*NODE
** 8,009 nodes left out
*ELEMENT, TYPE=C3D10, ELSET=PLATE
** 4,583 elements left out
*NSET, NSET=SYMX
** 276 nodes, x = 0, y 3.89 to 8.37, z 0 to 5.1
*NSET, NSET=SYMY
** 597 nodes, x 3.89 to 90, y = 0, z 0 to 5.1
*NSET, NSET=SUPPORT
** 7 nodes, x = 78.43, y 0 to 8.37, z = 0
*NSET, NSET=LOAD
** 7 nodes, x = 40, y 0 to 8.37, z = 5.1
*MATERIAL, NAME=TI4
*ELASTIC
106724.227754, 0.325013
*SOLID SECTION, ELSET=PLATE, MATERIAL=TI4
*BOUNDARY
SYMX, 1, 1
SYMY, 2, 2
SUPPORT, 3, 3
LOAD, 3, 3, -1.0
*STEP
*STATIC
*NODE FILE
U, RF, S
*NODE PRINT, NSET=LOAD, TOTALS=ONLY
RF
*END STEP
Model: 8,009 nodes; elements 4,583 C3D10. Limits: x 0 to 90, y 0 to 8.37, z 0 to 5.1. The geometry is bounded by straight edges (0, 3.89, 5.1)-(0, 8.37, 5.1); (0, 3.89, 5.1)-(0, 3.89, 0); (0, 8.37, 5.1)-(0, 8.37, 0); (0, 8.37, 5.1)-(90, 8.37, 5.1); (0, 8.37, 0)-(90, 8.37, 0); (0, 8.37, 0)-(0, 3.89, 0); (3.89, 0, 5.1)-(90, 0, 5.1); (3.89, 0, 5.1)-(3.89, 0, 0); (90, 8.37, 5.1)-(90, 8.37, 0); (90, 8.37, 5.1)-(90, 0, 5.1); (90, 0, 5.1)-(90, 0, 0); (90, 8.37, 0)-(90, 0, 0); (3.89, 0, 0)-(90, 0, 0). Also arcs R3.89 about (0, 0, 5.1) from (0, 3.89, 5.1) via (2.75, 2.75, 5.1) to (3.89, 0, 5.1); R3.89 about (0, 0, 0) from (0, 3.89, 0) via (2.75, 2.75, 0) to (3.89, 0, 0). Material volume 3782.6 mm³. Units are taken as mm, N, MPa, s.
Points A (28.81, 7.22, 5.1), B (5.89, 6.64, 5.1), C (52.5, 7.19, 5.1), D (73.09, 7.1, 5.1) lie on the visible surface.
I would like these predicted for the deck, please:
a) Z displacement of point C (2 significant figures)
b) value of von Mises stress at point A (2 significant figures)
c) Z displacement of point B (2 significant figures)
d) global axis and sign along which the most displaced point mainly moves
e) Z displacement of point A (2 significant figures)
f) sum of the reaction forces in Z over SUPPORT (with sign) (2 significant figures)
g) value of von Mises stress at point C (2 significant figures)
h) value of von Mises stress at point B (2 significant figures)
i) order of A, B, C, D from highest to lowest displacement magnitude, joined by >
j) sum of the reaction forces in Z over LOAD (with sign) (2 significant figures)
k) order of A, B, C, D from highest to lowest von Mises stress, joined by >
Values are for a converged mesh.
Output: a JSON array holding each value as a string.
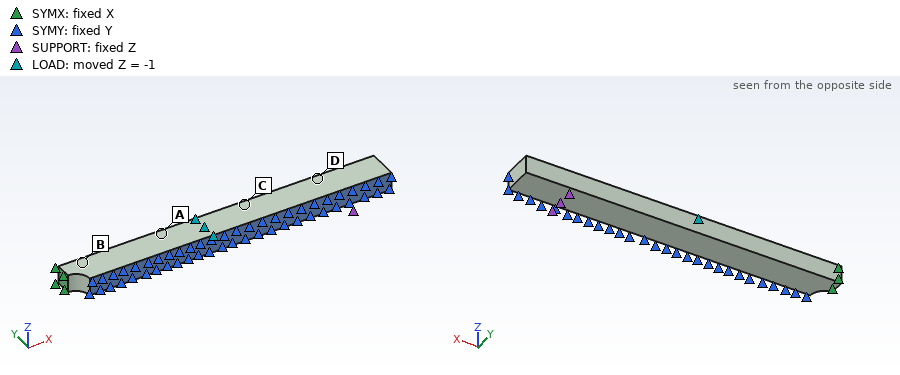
["-0.72 mm", "130 MPa", "-1.4 mm", "-Z", "-1.2 mm", "120 N", "85 MPa", "160 MPa", "B > A > C > D", "-120 N", "B > A > C > D"]
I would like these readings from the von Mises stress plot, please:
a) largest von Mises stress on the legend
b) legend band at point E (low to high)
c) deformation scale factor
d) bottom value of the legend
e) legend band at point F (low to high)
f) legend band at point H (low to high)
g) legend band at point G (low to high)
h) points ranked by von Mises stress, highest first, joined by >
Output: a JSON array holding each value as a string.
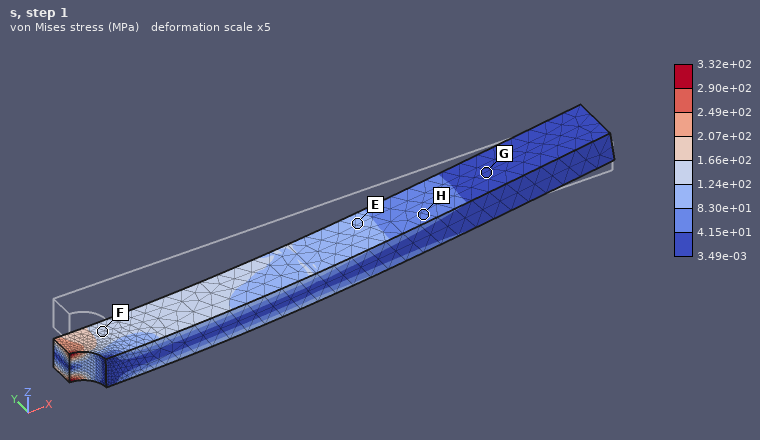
["3.32e+02 MPa", "8.30e+01 to 1.24e+02 MPa", "5", "3.49e-03 MPa", "1.24e+02 to 1.66e+02 MPa", "4.15e+01 to 8.30e+01 MPa", "3.49e-03 to 4.15e+01 MPa", "F > E > H > G"]
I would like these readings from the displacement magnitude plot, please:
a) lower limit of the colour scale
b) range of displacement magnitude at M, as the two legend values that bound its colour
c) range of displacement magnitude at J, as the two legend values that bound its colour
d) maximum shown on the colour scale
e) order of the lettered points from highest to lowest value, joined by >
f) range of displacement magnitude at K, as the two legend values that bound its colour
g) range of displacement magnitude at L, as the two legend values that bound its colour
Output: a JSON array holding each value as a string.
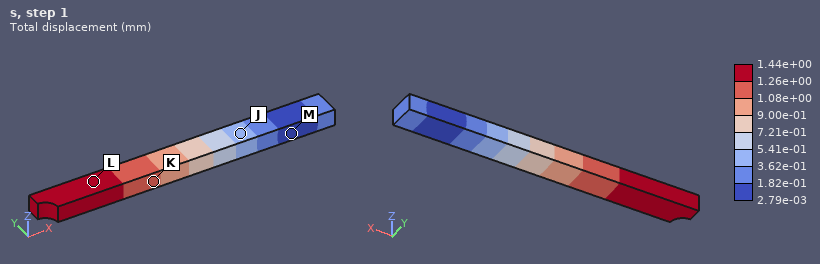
["2.79e-03 mm", "2.79e-03 to 1.82e-01 mm", "3.62e-01 to 5.41e-01 mm", "1.44e+00 mm", "L > K > J > M", "1.08e+00 to 1.26e+00 mm", "1.26e+00 to 1.44e+00 mm"]
